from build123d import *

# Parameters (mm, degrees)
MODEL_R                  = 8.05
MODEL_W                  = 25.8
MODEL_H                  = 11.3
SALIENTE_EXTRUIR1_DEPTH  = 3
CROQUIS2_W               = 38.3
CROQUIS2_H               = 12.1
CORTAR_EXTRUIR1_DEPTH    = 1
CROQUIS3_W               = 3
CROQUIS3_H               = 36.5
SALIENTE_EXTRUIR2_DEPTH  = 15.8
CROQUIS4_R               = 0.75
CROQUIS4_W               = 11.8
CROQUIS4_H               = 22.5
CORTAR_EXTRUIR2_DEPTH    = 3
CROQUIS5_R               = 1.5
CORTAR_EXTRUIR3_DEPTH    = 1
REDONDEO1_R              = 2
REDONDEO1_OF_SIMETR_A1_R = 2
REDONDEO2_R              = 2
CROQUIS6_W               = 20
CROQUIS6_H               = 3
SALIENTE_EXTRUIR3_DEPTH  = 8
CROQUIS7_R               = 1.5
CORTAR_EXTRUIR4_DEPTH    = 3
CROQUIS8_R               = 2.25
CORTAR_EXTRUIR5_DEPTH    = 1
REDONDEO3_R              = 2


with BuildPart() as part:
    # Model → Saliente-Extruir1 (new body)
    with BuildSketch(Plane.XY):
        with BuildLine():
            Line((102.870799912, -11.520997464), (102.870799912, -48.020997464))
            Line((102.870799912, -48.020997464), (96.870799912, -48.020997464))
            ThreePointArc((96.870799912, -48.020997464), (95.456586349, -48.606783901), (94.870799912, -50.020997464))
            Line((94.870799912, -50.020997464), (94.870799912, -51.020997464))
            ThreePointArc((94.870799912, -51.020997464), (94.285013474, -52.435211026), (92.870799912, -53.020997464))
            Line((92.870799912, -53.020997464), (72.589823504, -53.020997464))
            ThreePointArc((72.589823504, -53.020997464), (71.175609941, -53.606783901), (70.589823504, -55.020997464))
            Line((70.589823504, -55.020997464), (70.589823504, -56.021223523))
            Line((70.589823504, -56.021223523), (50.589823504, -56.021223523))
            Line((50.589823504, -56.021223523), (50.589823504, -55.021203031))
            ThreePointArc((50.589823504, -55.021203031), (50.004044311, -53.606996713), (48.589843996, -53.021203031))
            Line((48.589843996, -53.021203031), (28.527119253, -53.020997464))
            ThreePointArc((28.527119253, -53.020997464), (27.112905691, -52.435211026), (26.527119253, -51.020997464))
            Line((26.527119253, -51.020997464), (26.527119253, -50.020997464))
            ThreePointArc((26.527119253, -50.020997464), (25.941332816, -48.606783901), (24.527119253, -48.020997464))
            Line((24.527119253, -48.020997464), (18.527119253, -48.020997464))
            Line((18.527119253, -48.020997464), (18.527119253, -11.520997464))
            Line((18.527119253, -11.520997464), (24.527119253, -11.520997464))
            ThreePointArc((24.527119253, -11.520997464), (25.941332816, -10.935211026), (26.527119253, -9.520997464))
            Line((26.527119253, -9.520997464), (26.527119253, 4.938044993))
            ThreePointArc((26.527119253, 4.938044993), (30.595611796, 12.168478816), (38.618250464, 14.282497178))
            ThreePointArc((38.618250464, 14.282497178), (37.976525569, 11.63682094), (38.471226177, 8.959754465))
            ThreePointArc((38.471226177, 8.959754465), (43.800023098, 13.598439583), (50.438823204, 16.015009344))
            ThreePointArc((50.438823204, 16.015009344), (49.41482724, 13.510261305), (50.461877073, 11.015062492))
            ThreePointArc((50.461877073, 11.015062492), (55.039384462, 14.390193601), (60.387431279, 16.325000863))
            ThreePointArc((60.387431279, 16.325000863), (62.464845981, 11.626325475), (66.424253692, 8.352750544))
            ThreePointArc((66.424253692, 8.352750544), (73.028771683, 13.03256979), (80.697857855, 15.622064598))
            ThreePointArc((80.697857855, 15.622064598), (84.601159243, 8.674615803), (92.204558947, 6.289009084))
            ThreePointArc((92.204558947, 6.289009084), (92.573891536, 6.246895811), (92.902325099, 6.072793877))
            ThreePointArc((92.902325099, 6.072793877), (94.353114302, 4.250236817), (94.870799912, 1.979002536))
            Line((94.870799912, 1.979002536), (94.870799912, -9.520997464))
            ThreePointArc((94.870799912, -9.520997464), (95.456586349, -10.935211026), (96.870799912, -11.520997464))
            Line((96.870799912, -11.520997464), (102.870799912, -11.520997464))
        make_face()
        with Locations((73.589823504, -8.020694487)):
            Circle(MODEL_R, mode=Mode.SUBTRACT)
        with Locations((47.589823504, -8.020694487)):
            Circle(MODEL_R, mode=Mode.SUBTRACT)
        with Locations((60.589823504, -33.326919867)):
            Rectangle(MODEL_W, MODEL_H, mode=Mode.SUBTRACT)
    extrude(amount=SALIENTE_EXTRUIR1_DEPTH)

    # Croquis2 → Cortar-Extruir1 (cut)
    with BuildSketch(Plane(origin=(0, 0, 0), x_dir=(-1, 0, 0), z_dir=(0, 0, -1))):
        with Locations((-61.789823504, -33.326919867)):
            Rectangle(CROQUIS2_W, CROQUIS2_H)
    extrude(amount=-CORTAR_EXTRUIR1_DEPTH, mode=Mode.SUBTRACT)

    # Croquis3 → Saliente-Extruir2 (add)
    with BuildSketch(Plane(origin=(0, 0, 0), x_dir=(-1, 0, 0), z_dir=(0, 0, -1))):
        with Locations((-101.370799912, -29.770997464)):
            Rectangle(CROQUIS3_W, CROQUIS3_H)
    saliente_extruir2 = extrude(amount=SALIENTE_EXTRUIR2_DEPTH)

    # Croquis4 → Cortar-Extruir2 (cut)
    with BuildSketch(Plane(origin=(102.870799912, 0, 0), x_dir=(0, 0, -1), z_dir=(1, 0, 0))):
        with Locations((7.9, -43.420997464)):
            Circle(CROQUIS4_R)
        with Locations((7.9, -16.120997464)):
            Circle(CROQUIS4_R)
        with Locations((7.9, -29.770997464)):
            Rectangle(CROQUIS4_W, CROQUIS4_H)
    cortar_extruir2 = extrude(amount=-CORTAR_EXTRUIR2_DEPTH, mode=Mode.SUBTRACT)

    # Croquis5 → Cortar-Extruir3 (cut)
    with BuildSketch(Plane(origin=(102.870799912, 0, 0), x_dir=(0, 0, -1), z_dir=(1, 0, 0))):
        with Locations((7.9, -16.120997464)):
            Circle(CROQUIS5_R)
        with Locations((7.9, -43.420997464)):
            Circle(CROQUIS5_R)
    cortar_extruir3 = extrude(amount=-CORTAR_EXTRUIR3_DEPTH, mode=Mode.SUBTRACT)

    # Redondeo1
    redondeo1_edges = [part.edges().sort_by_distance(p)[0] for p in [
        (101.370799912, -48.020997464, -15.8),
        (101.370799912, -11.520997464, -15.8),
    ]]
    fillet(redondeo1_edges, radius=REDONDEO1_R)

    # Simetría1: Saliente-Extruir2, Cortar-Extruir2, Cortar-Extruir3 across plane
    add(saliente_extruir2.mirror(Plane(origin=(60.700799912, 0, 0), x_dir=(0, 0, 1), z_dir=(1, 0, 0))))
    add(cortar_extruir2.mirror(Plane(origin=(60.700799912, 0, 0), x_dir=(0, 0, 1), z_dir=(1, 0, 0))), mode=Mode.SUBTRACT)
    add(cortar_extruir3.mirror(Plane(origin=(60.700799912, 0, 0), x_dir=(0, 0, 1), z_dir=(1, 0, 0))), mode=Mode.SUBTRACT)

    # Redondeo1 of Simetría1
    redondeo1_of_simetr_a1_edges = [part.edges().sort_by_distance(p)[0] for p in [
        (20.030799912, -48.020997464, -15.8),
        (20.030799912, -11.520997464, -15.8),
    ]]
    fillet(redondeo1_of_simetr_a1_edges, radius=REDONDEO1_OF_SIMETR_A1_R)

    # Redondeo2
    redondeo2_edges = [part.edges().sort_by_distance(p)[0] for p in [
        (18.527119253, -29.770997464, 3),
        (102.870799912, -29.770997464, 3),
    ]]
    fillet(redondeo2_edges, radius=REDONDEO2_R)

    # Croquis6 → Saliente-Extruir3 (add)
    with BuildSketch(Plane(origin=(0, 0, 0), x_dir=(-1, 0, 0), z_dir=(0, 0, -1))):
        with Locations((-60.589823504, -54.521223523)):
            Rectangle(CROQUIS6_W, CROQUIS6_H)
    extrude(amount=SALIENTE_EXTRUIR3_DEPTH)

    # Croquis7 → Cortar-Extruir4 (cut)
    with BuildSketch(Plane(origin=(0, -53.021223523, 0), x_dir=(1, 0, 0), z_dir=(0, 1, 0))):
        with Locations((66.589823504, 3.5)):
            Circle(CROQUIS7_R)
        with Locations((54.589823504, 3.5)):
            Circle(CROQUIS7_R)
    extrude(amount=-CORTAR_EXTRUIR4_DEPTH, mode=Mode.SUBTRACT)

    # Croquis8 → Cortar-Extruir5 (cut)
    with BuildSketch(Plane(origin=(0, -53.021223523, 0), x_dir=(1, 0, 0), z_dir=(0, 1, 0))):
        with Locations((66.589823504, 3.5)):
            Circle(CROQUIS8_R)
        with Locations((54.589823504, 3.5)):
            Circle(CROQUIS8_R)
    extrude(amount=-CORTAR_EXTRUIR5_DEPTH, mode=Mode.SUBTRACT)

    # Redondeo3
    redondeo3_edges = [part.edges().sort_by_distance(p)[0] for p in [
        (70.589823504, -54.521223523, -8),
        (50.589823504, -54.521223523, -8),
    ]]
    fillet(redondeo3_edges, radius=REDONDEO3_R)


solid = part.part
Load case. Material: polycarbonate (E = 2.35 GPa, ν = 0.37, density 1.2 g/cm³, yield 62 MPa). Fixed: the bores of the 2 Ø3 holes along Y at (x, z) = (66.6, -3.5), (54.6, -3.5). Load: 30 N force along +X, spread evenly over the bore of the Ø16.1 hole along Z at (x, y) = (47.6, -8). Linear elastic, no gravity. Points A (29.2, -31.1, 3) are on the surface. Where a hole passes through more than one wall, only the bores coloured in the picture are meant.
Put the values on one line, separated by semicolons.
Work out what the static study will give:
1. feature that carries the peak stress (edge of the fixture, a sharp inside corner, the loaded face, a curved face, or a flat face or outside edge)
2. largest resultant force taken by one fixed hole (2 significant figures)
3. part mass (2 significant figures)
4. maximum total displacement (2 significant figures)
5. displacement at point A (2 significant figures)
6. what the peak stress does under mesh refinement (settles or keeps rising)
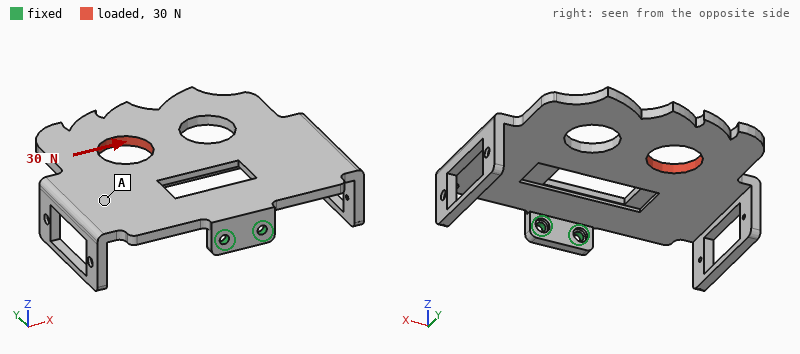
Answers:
edge of the fixture; 110 N; 18 g; 1.2 mm; 0.66 mm; keeps rising
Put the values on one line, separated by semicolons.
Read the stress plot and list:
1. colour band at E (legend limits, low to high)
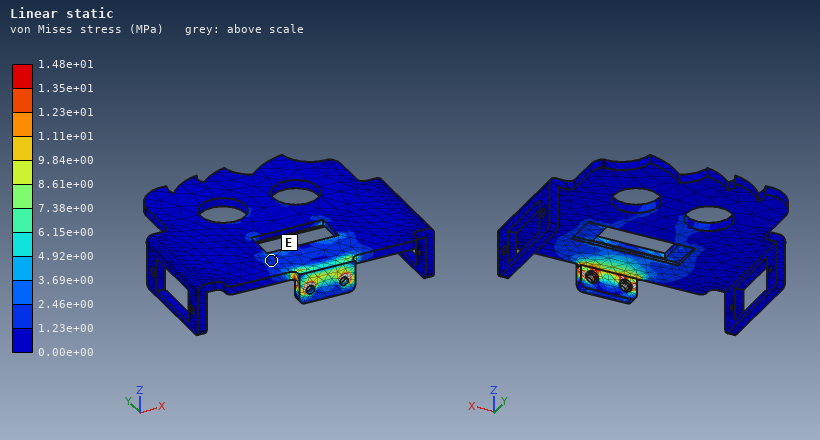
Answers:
1.23e+00 to 2.46e+00 MPa
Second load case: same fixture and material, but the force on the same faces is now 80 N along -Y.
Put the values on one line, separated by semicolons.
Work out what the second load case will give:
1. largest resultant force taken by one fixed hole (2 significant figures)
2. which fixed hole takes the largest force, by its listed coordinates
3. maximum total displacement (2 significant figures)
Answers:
120 N; (54.6, -3.5); 1.4 mm
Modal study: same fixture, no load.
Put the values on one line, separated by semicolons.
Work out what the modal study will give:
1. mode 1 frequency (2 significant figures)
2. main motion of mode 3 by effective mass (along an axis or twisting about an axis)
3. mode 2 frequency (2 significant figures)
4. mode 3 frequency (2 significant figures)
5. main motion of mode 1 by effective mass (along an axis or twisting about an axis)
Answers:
83 Hz; along X; 150 Hz; 270 Hz; along Z
